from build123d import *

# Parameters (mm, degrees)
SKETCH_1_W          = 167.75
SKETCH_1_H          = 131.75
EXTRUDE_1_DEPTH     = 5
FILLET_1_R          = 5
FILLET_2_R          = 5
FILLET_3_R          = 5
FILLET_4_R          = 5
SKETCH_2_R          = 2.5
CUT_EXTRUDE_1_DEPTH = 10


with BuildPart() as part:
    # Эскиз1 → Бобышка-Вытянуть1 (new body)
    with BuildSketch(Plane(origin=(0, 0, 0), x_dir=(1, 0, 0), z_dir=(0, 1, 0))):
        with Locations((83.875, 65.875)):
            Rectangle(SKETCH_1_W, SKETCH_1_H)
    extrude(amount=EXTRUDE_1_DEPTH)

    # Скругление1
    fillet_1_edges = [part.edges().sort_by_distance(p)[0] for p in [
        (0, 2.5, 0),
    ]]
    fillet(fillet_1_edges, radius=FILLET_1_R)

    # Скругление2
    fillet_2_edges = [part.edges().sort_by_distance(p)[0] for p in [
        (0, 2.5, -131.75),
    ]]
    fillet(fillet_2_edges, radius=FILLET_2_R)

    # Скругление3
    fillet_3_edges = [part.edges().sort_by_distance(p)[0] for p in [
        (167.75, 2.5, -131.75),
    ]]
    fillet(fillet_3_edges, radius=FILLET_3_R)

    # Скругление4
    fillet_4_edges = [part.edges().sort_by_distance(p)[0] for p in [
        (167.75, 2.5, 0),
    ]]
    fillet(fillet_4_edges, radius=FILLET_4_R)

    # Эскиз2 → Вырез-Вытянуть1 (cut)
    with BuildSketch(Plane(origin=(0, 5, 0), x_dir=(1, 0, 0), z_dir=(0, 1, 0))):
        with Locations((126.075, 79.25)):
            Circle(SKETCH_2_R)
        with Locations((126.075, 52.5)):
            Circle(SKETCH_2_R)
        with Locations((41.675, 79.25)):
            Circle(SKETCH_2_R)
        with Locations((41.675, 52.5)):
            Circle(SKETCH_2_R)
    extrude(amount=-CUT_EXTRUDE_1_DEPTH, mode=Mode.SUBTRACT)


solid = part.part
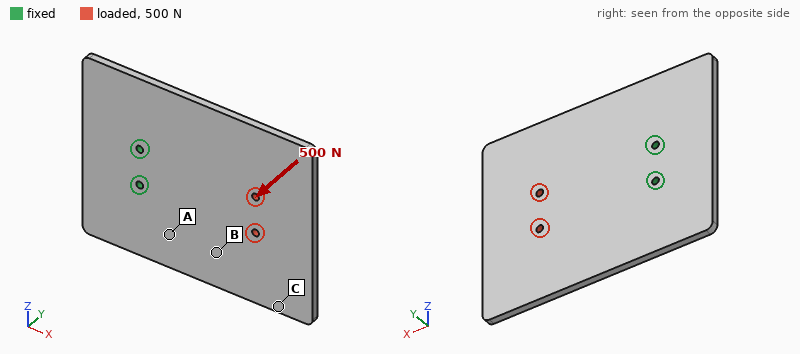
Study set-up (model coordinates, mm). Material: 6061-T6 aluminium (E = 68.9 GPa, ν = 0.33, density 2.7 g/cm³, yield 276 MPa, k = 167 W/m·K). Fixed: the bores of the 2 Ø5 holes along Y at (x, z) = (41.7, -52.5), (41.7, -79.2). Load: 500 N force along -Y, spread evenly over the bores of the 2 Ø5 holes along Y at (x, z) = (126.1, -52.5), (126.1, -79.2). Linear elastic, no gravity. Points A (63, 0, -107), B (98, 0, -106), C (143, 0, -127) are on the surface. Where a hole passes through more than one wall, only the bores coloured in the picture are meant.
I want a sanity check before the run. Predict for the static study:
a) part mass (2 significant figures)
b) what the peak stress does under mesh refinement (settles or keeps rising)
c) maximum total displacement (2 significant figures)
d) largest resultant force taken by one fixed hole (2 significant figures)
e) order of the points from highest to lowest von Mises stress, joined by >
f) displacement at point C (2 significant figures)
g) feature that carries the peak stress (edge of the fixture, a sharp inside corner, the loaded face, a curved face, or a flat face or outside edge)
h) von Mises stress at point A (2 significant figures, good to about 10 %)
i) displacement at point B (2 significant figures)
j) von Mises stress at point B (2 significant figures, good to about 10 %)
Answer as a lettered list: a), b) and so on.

a) 300 g
b) keeps rising
c) 2.3 mm
d) 250 N
e) A > B > C
f) 1.6 mm
g) edge of the fixture
h) 49 MPa
i) 0.73 mm
j) 26 MPa
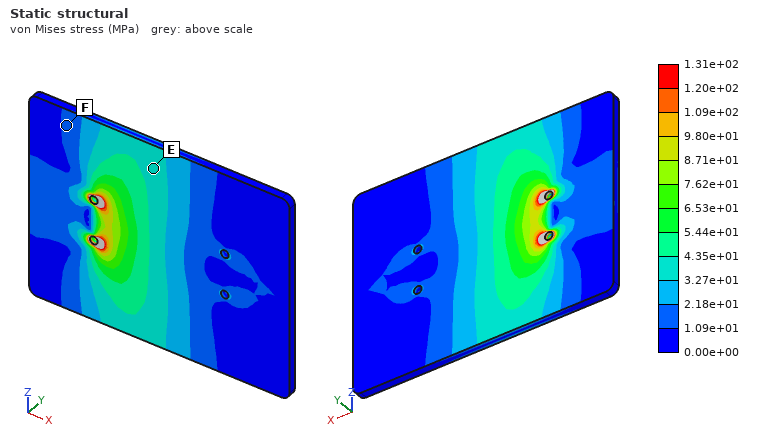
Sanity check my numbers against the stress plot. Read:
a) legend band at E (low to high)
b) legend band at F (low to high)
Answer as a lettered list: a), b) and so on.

a) 3.27e+01 to 4.35e+01 MPa
b) 1.09e+01 to 2.18e+01 MPa
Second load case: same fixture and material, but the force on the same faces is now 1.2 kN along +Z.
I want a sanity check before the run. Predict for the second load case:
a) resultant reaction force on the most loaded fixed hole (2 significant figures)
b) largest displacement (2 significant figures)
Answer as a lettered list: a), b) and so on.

a) 3.5 kN
b) 88 µm
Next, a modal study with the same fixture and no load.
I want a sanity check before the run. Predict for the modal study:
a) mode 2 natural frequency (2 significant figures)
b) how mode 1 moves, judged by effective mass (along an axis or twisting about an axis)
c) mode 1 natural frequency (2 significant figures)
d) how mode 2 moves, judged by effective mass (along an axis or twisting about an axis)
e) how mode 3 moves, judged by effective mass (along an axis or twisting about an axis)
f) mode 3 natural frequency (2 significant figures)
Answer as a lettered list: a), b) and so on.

a) 490 Hz
b) along Y
c) 230 Hz
d) twisting about X
e) along Y
f) 1200 Hz
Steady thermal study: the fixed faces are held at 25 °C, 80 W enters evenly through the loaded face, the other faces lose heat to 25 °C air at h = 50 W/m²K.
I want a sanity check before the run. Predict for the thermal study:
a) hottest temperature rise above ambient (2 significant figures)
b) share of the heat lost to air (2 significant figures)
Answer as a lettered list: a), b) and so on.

a) 55 K
b) 61 %
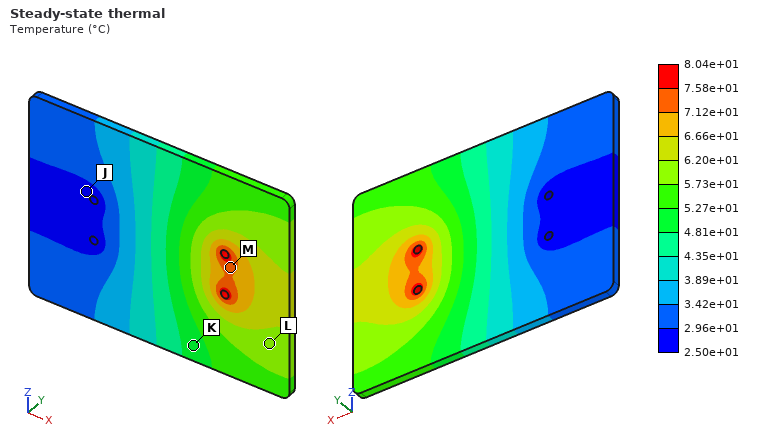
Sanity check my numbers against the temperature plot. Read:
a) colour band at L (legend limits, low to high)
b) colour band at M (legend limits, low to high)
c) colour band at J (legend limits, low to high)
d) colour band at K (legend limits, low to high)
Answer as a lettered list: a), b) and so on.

a) 5.73e+01 to 6.20e+01 °C
b) 7.12e+01 to 7.58e+01 °C
c) 2.50e+01 to 2.96e+01 °C
d) 4.81e+01 to 5.27e+01 °C
